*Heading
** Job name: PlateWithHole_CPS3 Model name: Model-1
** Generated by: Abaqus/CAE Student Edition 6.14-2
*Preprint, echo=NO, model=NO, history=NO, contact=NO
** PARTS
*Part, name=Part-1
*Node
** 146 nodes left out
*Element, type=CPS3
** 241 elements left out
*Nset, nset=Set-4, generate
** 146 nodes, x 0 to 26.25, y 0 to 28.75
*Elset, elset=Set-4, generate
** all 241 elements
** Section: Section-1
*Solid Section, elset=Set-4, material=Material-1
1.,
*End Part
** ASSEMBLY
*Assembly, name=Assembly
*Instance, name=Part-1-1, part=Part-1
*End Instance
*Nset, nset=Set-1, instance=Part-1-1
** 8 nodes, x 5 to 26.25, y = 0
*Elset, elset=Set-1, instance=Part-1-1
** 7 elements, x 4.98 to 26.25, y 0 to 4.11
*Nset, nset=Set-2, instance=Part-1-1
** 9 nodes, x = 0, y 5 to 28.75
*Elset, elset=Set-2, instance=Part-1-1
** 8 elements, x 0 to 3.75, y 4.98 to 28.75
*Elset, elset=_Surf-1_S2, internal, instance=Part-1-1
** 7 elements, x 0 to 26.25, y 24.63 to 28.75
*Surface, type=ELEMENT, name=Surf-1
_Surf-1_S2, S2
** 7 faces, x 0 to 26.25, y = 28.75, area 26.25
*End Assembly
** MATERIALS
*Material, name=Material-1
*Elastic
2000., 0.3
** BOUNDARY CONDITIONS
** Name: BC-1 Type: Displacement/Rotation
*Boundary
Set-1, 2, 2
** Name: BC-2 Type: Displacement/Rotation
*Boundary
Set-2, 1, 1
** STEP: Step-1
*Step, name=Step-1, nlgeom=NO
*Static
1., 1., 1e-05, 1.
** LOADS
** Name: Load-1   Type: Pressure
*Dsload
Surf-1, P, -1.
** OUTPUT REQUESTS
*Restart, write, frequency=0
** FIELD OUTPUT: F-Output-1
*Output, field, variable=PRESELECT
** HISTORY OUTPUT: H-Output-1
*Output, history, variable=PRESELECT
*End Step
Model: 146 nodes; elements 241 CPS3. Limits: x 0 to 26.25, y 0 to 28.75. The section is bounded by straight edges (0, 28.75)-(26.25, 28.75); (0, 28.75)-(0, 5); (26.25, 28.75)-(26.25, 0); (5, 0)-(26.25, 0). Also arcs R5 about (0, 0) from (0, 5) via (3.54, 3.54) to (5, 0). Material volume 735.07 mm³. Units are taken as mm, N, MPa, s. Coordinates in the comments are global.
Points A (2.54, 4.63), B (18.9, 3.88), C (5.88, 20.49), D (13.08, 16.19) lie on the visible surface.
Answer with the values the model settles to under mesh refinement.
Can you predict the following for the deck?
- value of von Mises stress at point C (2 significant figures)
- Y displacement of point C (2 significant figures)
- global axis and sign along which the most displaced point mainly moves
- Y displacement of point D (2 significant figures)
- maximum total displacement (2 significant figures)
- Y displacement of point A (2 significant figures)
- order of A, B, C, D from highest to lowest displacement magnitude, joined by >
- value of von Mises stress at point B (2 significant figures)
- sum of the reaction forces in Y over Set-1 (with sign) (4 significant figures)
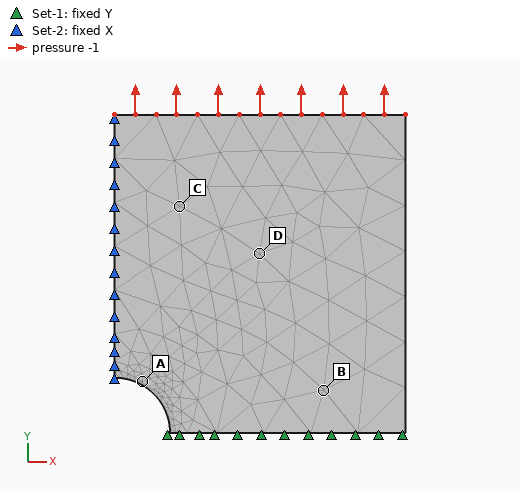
0.96 MPa
0.013 mm
+Y
0.0093 mm
0.017 mm
0.0071 mm
C > D > A > B
1.0 MPa
-26.25 N
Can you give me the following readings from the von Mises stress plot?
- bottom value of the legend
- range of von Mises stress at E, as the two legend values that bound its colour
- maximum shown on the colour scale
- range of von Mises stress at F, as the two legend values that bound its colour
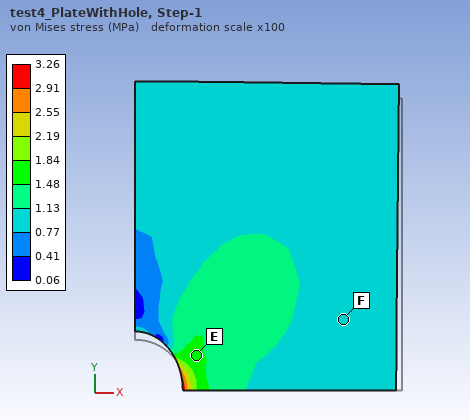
0.06 MPa
1.48 to 1.84 MPa
3.26 MPa
0.77 to 1.13 MPa
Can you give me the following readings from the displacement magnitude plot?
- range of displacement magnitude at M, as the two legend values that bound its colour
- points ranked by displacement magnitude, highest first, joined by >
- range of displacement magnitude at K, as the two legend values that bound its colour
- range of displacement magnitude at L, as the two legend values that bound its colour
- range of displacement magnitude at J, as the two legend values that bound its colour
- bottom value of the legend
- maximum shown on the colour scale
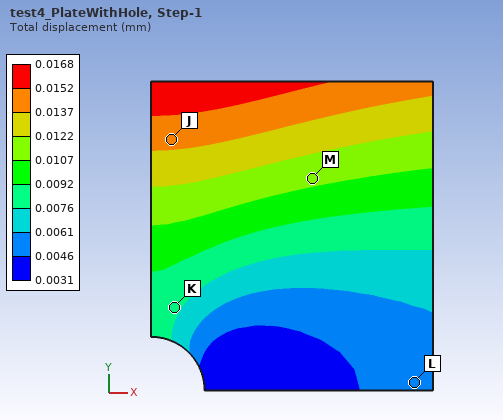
0.0107 to 0.0122 mm
J > M > K > L
0.0076 to 0.0092 mm
0.0046 to 0.0061 mm
0.0137 to 0.0152 mm
0.0031 mm
0.0168 mm
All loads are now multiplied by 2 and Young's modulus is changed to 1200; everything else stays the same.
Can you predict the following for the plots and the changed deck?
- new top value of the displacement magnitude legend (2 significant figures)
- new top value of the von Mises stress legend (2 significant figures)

0.056 mm
6.5 MPa
